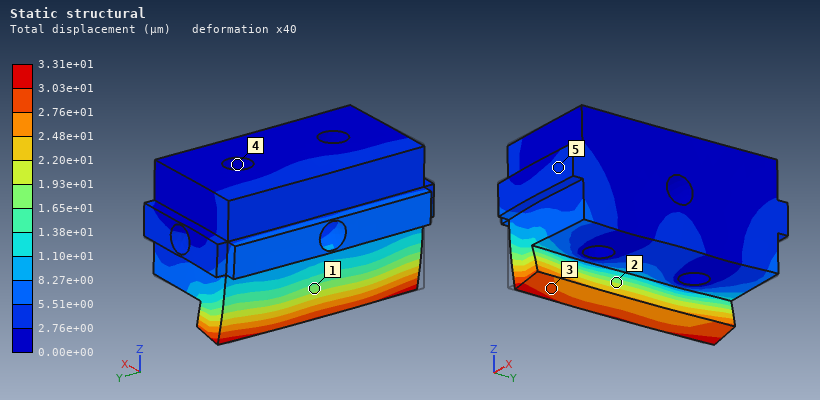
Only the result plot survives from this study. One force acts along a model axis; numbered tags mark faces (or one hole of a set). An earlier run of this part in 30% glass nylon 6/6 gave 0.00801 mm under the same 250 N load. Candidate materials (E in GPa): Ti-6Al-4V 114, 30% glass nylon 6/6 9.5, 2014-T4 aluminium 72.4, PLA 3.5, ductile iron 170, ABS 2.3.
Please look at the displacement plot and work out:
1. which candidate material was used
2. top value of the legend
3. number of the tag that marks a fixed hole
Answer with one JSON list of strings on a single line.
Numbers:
["ABS", "3.31e+01 µm", "4"]
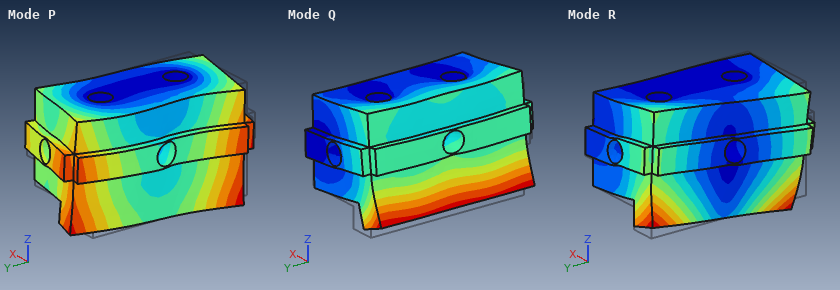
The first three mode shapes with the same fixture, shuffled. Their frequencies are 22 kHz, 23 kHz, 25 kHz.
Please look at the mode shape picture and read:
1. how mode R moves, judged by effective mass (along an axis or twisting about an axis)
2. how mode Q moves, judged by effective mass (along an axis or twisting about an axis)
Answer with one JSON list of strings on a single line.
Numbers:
["twisting about X", "along Z"]
